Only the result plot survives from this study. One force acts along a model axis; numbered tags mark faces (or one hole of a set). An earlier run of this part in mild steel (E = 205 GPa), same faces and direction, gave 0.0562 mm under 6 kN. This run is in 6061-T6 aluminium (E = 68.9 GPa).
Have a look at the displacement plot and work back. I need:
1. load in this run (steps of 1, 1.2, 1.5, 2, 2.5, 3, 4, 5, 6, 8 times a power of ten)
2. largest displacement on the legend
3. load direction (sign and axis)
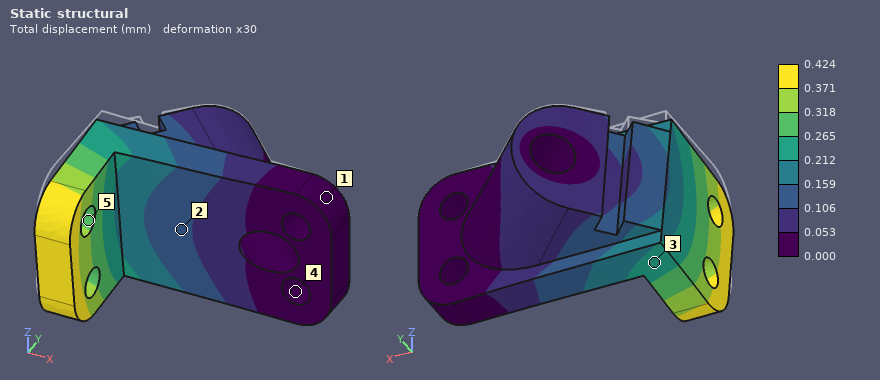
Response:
15 kN
0.424 mm
-Z
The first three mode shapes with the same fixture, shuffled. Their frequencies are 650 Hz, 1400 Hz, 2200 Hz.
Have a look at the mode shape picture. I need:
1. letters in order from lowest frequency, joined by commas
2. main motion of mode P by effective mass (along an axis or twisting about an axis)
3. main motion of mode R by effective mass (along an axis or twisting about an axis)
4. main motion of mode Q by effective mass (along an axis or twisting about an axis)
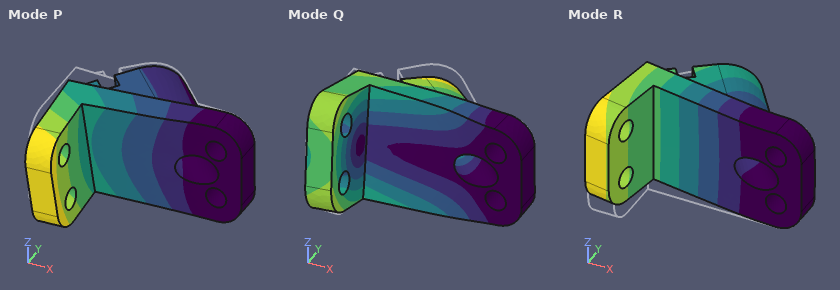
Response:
R, P, Q
along Z
along Y
along Z
